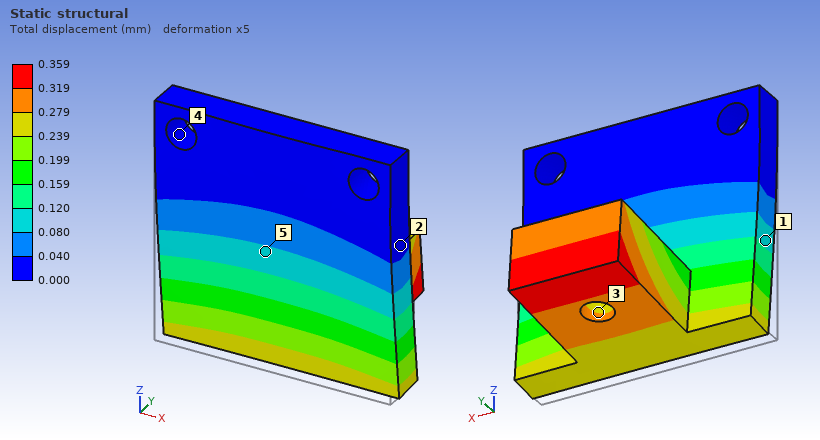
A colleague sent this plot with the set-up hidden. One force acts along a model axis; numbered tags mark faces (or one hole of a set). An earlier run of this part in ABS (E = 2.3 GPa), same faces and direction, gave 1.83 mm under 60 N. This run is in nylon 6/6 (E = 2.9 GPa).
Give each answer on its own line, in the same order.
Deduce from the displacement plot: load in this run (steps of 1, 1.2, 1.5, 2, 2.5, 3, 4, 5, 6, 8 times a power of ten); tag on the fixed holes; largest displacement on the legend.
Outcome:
15 N
4
0.359 mm
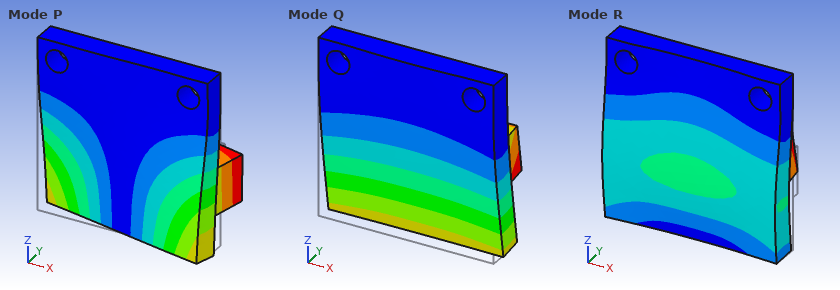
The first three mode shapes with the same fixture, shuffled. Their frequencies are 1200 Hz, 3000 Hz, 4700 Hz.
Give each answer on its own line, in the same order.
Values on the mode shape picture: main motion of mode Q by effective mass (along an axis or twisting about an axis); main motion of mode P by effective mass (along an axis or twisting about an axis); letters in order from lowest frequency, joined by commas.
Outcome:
along Y
along X
Q, P, R
